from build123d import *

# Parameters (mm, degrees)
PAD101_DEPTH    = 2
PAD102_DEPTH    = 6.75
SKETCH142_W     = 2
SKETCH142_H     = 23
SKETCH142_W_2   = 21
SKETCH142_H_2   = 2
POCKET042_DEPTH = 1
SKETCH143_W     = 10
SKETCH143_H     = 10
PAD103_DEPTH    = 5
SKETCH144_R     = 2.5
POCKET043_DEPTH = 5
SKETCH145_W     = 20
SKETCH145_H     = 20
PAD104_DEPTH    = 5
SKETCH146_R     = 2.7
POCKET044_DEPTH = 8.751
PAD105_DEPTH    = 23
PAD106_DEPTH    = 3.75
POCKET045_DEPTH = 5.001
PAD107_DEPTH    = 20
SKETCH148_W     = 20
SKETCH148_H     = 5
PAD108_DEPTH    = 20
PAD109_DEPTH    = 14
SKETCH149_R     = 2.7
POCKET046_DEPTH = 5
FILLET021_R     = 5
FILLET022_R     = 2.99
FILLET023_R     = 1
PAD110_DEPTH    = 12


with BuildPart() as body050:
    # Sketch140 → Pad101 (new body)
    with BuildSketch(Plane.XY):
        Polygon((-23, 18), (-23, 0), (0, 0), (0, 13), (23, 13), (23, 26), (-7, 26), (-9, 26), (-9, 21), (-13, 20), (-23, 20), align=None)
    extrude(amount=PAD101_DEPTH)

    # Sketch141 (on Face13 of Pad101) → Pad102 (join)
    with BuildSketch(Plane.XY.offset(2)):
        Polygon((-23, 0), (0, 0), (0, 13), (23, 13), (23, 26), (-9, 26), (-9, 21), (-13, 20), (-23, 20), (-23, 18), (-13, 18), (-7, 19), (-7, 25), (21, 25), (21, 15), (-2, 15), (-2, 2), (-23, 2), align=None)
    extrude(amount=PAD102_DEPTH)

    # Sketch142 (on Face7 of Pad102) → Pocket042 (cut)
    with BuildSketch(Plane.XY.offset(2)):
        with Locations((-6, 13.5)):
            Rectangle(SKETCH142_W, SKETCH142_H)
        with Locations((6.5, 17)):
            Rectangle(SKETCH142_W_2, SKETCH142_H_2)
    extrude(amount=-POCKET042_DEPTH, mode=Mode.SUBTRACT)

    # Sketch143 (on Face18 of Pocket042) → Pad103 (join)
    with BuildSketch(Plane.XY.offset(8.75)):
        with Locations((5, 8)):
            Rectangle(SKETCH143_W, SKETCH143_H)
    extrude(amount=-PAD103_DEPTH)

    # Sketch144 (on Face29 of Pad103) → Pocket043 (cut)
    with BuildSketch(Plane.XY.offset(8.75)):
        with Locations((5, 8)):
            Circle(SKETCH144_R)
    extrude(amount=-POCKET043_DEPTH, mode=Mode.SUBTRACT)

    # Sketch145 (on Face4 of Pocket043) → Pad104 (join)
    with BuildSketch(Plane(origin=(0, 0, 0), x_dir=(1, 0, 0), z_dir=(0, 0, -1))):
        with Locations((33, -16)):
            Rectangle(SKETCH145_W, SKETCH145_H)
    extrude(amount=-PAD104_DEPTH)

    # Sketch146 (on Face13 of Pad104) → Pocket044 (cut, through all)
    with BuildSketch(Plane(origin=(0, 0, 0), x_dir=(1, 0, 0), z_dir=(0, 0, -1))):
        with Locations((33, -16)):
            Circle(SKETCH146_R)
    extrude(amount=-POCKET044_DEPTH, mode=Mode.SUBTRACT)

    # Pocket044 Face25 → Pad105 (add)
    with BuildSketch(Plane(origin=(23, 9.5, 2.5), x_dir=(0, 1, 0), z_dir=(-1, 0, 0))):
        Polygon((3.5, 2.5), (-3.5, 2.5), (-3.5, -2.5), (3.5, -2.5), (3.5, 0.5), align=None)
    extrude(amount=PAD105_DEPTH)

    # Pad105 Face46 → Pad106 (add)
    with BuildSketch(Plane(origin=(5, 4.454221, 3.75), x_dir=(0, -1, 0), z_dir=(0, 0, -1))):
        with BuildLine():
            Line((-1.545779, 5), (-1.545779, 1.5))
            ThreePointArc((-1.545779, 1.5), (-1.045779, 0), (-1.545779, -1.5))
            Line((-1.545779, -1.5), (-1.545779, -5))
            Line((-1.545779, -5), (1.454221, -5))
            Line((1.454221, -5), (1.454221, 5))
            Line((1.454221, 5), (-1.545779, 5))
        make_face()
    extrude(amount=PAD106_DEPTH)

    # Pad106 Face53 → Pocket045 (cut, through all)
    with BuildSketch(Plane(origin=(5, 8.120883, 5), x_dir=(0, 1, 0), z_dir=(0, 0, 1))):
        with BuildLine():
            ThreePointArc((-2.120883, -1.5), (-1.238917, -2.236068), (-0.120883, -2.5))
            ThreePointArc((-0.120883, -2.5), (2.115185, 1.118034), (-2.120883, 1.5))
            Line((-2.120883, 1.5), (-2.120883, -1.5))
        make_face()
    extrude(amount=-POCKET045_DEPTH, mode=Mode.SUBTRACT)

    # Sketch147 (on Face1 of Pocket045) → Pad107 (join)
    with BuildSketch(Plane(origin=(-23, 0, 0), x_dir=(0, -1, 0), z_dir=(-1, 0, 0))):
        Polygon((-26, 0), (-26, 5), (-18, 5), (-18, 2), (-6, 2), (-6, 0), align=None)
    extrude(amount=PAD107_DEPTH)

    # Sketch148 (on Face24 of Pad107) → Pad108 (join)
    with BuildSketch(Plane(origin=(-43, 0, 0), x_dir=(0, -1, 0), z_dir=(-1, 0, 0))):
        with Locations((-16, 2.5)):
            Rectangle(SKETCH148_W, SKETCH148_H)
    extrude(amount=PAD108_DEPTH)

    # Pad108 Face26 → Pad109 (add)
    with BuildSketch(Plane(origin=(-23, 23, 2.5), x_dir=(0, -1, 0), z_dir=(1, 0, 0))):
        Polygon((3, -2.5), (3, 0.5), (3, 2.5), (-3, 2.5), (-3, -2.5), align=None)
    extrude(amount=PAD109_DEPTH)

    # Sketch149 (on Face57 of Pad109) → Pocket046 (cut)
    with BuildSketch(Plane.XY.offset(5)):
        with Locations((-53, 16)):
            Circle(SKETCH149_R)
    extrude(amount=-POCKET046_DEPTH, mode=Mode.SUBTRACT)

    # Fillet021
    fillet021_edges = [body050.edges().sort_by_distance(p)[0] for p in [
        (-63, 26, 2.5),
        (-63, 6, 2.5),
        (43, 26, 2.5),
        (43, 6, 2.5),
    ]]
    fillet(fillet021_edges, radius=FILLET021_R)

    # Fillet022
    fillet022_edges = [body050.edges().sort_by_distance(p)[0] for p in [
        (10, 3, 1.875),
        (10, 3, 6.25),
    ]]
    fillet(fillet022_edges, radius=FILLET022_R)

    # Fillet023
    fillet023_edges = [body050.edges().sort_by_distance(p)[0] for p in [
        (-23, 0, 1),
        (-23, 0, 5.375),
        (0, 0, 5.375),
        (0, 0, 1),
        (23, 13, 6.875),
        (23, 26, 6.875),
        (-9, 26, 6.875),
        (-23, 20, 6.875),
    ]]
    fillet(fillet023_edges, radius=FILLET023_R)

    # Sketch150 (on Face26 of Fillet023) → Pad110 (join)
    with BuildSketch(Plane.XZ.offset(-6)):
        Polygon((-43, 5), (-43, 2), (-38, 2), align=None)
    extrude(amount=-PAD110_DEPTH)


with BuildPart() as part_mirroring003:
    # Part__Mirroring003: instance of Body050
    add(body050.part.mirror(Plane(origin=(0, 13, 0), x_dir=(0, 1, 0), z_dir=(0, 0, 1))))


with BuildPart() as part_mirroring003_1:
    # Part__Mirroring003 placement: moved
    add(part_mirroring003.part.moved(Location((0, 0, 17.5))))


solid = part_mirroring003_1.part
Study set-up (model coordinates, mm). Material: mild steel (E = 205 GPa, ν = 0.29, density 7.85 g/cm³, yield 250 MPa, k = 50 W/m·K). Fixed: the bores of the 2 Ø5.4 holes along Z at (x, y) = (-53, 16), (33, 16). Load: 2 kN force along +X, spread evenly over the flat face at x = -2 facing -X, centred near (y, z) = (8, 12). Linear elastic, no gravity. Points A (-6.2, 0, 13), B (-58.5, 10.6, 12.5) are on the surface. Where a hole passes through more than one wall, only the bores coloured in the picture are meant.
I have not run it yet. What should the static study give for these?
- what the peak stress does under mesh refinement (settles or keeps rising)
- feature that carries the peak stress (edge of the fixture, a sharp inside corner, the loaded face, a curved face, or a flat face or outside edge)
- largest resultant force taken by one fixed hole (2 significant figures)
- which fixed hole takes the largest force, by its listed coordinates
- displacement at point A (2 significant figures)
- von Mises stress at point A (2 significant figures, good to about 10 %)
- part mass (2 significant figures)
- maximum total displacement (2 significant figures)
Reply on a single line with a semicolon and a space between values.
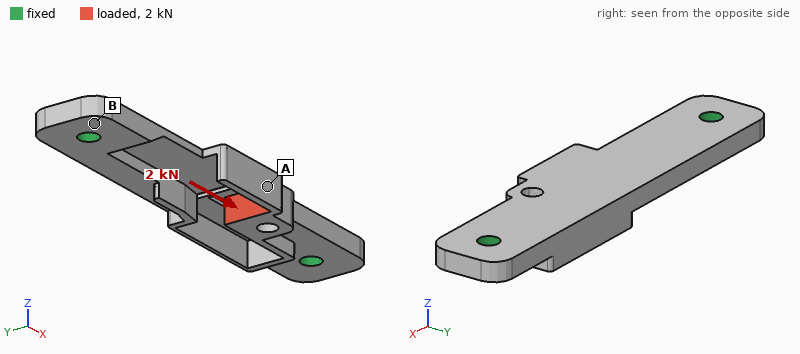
keeps rising; a sharp inside corner; 1.7 kN; (33, 16); 31 µm; 22 MPa; 75 g; 50 µm
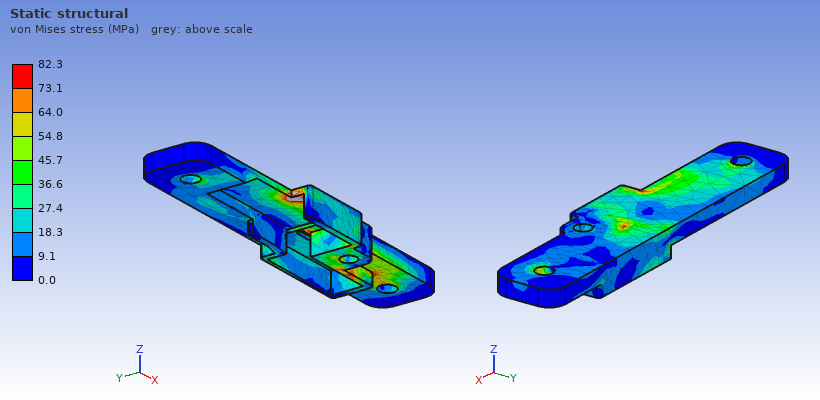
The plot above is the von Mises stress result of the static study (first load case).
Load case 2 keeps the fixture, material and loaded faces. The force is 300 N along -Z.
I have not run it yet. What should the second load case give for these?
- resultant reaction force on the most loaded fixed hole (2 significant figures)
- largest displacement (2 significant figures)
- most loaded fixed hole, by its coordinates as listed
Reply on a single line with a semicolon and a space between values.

300 N; 56 µm; (33, 16)
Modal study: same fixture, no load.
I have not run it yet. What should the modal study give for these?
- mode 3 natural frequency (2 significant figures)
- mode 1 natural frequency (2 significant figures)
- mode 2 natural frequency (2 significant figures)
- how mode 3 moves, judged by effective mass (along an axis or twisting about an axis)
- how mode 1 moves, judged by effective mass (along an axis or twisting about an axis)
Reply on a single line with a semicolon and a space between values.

8200 Hz; 3100 Hz; 5200 Hz; along Y; along Z
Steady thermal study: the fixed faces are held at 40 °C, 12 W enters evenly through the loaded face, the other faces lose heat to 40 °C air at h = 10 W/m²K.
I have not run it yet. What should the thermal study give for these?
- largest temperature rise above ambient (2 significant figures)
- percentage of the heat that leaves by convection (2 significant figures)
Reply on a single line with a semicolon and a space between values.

71 K; 14 %
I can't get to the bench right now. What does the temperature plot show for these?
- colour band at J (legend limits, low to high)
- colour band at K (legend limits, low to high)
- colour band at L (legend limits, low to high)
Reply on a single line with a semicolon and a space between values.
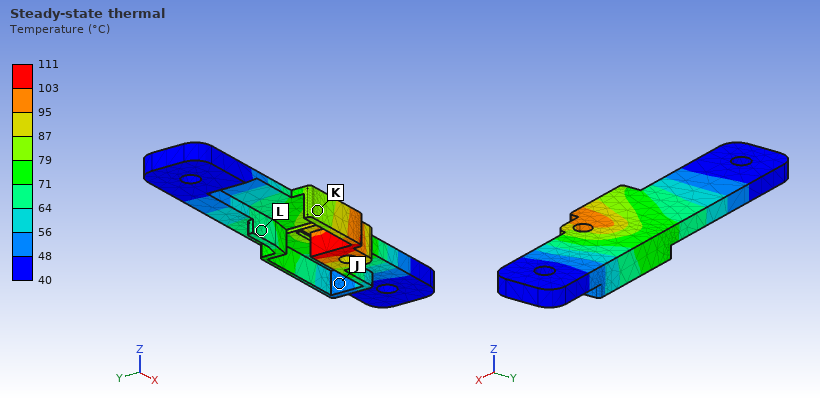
48 to 56 °C; 79 to 87 °C; 64 to 71 °C
